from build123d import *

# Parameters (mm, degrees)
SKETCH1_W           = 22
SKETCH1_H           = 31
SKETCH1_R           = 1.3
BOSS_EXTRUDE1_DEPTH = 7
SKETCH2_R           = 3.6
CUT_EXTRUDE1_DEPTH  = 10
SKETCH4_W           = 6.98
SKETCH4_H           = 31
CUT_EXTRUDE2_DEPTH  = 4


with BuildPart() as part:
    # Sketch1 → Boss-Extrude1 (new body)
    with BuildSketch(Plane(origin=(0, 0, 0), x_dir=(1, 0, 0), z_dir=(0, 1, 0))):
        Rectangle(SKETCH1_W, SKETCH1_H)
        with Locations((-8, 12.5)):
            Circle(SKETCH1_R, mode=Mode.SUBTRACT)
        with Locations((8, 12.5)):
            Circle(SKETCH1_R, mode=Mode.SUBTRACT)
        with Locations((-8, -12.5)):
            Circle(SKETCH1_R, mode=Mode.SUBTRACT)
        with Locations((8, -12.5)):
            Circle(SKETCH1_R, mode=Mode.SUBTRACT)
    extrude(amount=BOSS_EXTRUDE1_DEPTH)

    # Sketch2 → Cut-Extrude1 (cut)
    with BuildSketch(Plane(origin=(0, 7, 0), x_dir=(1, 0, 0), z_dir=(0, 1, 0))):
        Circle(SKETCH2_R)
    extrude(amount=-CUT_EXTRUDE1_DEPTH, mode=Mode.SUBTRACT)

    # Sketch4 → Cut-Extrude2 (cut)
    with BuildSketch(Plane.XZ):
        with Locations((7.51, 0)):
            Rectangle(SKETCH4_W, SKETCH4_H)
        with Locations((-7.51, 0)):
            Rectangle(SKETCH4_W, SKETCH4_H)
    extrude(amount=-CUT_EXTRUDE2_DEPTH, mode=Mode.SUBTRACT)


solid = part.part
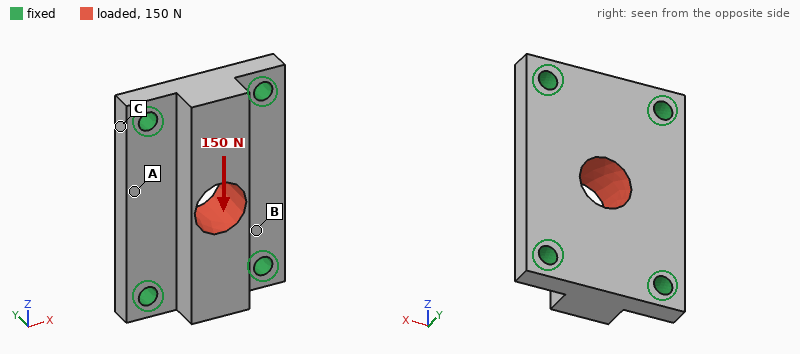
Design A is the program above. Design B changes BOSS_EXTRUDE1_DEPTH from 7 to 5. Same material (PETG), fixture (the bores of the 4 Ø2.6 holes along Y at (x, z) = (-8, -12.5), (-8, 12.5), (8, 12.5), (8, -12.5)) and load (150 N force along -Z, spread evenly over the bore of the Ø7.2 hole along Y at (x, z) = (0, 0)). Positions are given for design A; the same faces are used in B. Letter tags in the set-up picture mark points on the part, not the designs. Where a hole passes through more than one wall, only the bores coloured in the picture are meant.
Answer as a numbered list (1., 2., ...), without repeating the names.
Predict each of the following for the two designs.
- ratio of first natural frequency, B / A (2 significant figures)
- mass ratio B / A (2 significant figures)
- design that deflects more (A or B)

1. 0.54
2. 0.54
3. B
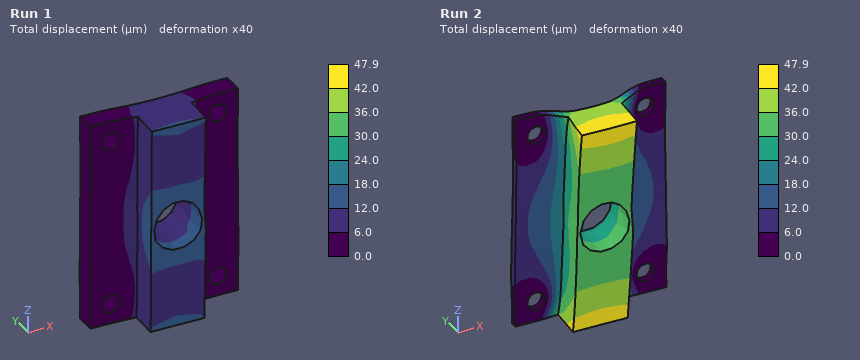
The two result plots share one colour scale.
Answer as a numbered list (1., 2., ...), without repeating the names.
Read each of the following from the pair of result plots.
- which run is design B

1. Run 2
